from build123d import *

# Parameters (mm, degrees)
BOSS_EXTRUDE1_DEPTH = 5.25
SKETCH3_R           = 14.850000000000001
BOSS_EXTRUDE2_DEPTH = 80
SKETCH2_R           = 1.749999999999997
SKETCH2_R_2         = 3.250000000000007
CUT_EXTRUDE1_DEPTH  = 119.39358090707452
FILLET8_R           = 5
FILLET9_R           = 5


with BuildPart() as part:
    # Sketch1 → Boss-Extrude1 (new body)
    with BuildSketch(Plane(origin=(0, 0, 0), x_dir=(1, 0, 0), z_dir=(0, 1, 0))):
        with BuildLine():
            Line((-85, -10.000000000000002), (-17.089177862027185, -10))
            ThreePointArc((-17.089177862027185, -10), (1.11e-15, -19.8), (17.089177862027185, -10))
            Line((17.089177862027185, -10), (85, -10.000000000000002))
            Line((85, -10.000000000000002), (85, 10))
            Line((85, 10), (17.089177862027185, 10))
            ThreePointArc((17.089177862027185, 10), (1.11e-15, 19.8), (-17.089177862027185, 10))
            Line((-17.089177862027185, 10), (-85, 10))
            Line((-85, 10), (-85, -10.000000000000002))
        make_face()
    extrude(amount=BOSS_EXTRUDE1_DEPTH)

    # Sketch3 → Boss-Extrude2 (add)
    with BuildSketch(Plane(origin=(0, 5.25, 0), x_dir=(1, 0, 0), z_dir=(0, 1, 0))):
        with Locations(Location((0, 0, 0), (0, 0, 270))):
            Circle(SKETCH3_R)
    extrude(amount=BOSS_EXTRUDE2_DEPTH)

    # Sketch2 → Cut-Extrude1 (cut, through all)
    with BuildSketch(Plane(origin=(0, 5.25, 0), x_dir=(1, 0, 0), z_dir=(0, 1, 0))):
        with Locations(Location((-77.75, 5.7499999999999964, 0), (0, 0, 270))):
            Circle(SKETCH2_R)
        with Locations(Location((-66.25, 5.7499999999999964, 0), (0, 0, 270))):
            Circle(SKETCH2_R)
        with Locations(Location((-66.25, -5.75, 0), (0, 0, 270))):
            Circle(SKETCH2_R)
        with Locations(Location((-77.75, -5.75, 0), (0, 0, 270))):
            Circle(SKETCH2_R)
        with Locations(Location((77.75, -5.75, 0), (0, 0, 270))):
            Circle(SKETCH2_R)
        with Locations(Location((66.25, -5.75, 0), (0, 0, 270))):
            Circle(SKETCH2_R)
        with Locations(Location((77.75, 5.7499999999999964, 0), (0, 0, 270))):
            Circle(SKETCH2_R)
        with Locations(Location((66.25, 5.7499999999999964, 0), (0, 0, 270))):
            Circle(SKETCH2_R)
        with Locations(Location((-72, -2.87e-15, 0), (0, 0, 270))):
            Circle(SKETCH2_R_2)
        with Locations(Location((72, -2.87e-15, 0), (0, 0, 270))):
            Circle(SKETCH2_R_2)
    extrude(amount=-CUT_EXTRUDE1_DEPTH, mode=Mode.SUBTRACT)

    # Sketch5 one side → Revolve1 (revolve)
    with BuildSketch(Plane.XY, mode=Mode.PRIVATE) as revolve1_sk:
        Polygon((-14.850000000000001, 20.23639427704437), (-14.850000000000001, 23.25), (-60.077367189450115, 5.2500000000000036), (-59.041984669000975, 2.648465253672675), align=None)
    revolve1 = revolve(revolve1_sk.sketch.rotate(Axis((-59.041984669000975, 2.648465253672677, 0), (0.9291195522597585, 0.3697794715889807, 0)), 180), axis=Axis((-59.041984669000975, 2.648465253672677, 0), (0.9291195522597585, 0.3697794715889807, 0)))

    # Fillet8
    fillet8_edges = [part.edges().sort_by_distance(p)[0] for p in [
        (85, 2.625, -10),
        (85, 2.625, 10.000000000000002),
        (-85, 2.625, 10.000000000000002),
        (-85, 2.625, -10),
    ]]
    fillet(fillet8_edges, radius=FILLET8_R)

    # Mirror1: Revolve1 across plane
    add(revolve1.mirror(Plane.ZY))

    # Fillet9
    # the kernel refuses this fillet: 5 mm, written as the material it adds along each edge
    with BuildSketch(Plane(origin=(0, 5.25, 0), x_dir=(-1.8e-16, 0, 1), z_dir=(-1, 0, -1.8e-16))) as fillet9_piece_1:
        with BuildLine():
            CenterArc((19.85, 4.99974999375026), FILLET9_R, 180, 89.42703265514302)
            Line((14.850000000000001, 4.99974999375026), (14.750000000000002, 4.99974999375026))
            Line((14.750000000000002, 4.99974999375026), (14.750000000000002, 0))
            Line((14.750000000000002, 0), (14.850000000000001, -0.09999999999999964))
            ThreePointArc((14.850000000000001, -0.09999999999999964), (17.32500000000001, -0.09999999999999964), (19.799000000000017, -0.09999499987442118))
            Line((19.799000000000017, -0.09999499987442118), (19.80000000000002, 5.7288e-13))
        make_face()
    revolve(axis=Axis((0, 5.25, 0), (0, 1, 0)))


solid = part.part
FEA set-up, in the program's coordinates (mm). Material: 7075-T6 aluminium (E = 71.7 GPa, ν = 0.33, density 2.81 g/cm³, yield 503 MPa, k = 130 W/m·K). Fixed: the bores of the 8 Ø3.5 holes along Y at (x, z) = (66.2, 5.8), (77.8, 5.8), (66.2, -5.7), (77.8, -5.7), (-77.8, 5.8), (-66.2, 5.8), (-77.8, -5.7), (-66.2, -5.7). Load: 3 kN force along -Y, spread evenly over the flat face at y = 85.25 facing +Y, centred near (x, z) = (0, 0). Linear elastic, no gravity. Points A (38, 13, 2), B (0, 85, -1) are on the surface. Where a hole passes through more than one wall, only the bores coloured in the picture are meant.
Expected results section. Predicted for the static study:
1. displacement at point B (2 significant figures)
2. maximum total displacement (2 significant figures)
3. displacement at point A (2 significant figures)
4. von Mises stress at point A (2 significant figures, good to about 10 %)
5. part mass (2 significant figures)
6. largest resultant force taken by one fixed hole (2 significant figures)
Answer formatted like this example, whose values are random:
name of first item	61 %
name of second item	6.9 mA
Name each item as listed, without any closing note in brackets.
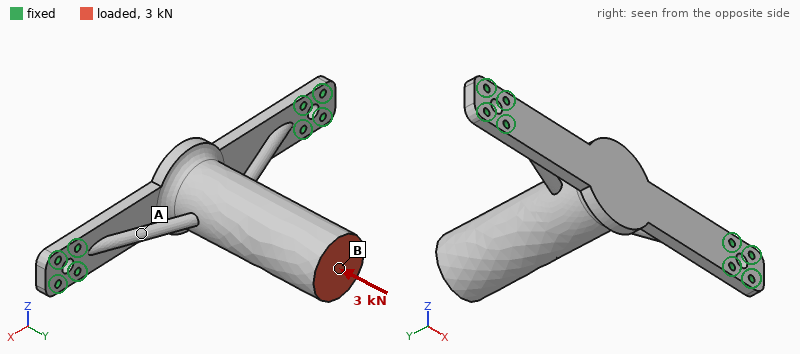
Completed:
displacement at point B	0.24 mm
maximum total displacement	0.24 mm
displacement at point A	0.14 mm
von Mises stress at point A	130 MPa
part mass	220 g
largest resultant force taken by one fixed hole	1.4 kN
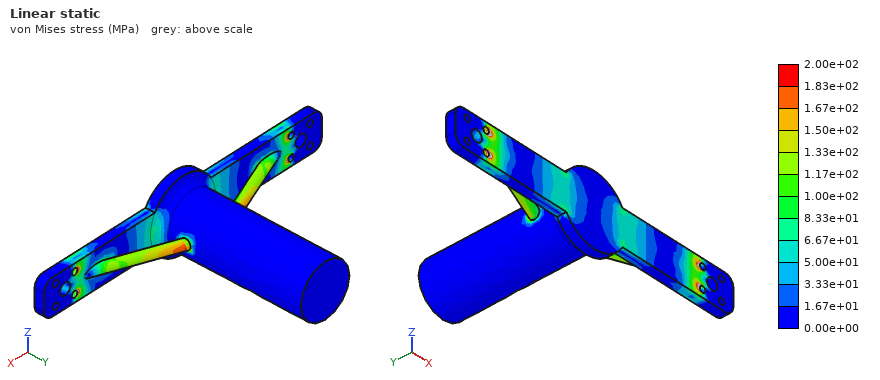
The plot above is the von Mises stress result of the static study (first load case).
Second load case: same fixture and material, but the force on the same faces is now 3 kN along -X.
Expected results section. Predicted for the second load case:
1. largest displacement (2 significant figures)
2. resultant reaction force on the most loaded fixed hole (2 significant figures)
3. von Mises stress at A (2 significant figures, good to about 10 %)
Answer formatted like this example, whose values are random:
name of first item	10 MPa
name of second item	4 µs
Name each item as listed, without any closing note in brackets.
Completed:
largest displacement	0.68 mm
resultant reaction force on the most loaded fixed hole	1.4 kN
von Mises stress at A	210 MPa
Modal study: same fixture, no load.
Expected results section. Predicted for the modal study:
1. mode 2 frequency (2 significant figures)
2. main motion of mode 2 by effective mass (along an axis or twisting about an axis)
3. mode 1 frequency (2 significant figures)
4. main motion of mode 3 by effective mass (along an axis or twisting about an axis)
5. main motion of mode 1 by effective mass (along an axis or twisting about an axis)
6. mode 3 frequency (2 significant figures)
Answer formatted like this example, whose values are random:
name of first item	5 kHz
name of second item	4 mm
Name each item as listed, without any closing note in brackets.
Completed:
mode 2 frequency	1300 Hz
main motion of mode 2 by effective mass	along Y
mode 1 frequency	280 Hz
main motion of mode 3 by effective mass	along X
main motion of mode 1 by effective mass	along Z
mode 3 frequency	1500 Hz
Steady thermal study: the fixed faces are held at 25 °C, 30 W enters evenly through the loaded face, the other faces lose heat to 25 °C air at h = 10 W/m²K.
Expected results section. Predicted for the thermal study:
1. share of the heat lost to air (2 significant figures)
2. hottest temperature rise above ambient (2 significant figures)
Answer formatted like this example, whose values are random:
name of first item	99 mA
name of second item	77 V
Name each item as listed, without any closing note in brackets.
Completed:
share of the heat lost to air	20 %
hottest temperature rise above ambient	65 K
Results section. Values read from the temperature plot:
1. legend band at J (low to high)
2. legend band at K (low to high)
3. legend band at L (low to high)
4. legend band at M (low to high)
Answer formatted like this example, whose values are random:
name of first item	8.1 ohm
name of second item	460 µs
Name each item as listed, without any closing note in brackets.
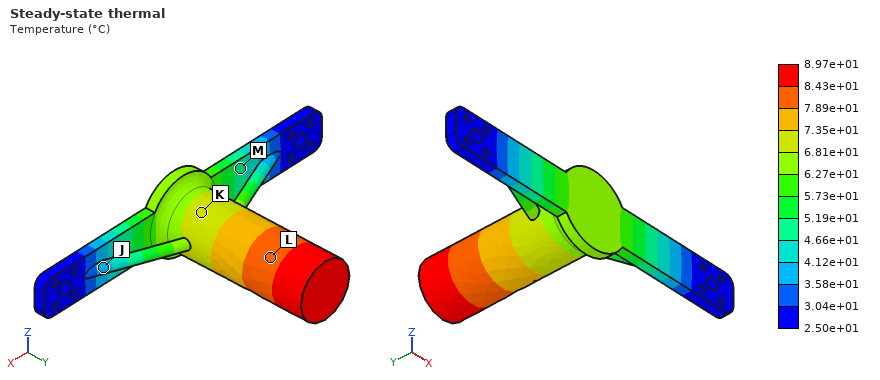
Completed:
legend band at J	3.58e+01 to 4.12e+01 °C
legend band at K	6.81e+01 to 7.35e+01 °C
legend band at L	7.89e+01 to 8.43e+01 °C
legend band at M	4.66e+01 to 5.19e+01 °C
